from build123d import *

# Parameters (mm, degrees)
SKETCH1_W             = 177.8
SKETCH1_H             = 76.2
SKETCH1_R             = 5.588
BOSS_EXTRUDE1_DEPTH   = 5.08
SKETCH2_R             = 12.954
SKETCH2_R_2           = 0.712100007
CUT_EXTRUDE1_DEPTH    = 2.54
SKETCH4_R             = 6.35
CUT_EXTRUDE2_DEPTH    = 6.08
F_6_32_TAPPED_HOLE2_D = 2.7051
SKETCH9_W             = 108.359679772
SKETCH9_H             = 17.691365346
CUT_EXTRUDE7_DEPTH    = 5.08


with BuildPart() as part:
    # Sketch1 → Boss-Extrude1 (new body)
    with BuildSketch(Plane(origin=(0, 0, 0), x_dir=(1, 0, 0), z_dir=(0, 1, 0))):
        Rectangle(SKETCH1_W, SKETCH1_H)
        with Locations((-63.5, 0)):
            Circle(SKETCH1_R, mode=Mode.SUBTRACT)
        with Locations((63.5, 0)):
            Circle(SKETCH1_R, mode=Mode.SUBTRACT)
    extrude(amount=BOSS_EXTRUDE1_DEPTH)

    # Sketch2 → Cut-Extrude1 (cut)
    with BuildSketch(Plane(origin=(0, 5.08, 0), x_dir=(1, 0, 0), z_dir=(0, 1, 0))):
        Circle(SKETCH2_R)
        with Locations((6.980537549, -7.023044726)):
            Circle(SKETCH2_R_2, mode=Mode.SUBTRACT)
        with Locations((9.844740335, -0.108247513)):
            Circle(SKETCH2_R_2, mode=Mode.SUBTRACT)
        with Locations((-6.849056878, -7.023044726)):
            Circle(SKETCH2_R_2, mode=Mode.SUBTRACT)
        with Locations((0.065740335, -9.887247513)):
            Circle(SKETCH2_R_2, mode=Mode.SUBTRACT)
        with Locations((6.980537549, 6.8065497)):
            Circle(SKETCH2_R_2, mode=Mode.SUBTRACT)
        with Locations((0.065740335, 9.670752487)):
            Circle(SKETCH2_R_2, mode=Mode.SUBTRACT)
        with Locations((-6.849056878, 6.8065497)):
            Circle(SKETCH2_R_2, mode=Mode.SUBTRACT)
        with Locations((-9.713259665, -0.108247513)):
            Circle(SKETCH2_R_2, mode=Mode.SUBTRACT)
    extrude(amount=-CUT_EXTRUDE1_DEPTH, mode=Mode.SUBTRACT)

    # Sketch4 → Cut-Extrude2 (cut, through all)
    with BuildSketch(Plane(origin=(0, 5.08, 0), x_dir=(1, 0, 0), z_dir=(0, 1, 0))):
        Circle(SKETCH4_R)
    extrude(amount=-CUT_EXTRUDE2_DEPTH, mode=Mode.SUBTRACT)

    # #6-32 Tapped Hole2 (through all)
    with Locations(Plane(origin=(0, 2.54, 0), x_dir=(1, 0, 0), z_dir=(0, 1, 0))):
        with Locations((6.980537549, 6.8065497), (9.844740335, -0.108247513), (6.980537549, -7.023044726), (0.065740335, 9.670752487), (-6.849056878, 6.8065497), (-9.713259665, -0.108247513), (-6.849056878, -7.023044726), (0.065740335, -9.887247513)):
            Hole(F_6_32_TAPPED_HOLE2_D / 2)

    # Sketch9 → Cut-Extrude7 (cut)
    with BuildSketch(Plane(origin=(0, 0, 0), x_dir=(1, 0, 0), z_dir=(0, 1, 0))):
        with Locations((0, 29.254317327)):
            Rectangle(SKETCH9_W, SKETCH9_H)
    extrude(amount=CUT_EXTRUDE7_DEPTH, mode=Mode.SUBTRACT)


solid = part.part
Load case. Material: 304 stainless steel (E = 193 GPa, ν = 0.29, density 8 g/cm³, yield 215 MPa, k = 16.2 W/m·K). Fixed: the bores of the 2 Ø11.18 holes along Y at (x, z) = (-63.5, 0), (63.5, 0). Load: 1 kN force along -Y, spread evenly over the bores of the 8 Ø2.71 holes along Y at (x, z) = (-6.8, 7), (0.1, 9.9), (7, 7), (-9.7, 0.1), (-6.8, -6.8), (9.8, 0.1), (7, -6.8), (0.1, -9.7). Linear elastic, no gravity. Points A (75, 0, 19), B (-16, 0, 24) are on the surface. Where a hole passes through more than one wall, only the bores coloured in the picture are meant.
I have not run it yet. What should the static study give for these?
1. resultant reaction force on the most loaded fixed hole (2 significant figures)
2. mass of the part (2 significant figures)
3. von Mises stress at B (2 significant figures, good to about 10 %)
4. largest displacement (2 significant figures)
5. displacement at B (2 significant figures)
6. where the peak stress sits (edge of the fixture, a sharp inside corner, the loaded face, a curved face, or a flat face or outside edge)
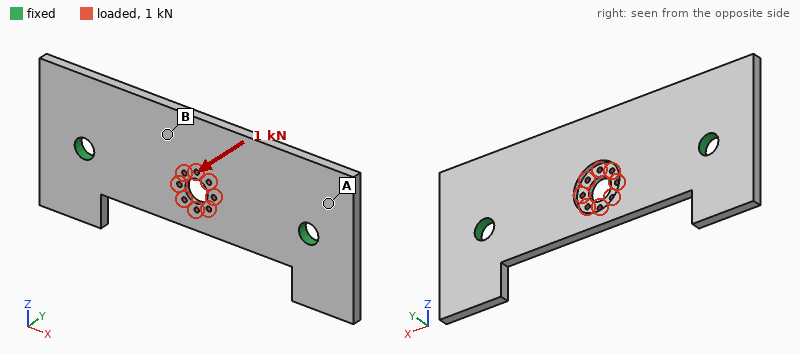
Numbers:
620 N
450 g
33 MPa
0.12 mm
0.070 mm
the loaded face
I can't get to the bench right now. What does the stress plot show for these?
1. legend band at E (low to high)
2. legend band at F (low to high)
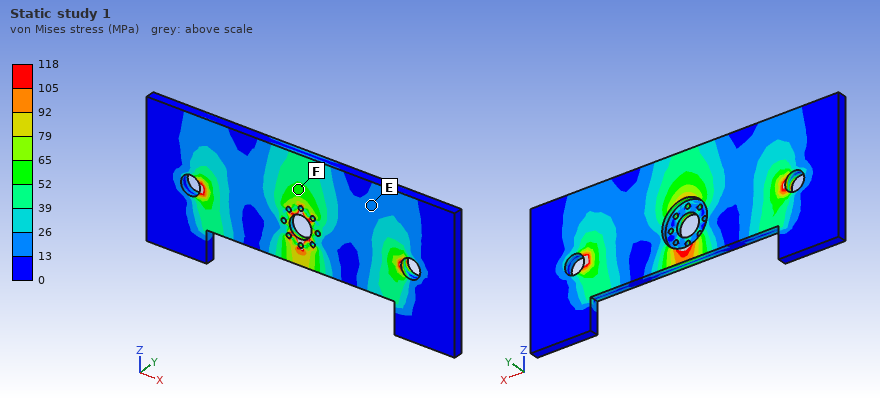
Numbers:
13 to 26 MPa
52 to 65 MPa
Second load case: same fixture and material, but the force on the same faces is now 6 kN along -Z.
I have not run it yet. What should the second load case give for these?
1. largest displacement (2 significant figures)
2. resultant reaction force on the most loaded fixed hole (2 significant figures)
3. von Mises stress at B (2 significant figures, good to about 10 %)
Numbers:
36 µm
3.3 kN
30 MPa
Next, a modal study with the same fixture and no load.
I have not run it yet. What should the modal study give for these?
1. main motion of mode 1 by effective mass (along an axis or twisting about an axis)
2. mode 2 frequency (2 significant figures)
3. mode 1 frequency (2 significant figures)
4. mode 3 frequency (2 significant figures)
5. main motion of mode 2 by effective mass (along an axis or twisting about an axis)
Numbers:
along Y
2300 Hz
1500 Hz
3000 Hz
twisting about X
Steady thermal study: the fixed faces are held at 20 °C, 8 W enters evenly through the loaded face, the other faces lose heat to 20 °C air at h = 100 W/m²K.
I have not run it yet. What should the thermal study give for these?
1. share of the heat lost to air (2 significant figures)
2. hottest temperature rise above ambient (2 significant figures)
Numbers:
94 %
27 K
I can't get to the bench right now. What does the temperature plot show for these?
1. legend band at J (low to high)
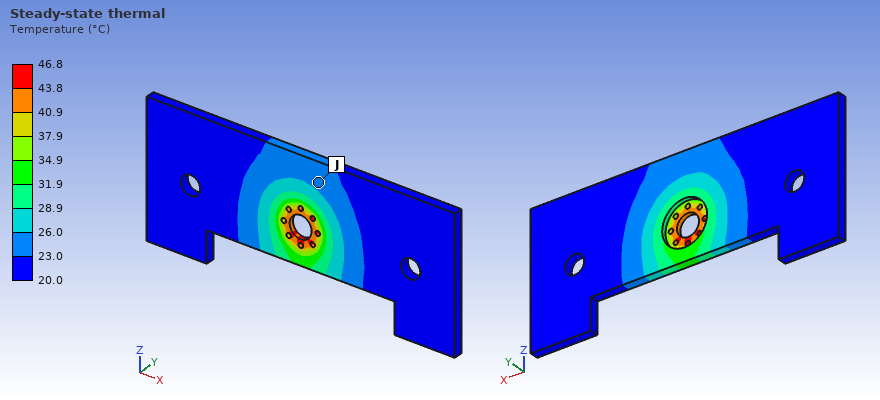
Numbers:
23.0 to 26.0 °C
